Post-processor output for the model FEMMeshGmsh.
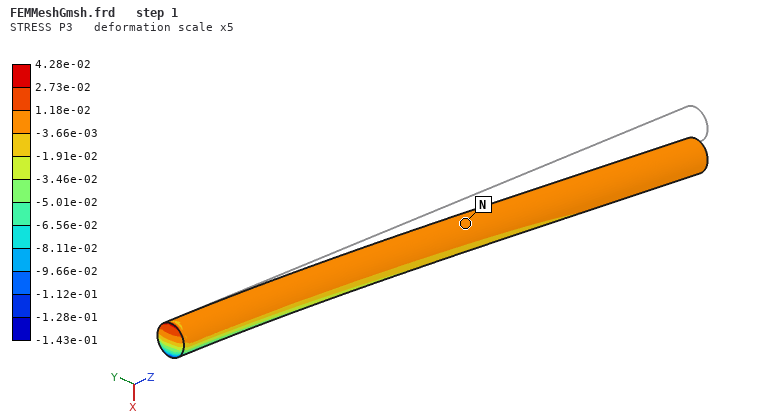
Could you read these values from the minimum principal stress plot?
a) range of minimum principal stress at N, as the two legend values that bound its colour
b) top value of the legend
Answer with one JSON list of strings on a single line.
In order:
["-3.66e-03 to 1.18e-02", "4.28e-02"]
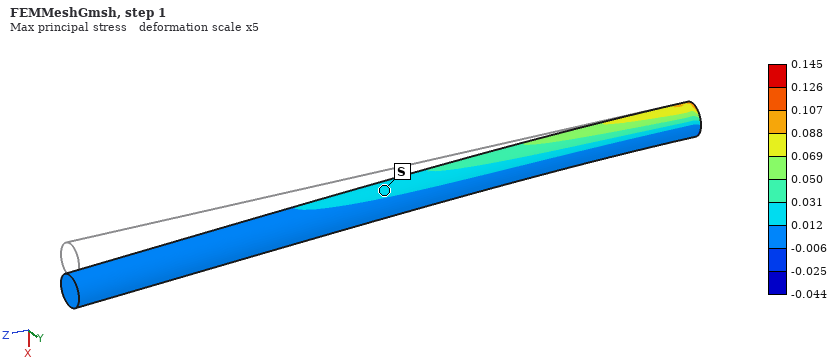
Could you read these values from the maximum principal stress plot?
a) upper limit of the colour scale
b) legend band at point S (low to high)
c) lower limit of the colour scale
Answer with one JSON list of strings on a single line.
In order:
["0.145", "0.012 to 0.031", "-0.044"]
